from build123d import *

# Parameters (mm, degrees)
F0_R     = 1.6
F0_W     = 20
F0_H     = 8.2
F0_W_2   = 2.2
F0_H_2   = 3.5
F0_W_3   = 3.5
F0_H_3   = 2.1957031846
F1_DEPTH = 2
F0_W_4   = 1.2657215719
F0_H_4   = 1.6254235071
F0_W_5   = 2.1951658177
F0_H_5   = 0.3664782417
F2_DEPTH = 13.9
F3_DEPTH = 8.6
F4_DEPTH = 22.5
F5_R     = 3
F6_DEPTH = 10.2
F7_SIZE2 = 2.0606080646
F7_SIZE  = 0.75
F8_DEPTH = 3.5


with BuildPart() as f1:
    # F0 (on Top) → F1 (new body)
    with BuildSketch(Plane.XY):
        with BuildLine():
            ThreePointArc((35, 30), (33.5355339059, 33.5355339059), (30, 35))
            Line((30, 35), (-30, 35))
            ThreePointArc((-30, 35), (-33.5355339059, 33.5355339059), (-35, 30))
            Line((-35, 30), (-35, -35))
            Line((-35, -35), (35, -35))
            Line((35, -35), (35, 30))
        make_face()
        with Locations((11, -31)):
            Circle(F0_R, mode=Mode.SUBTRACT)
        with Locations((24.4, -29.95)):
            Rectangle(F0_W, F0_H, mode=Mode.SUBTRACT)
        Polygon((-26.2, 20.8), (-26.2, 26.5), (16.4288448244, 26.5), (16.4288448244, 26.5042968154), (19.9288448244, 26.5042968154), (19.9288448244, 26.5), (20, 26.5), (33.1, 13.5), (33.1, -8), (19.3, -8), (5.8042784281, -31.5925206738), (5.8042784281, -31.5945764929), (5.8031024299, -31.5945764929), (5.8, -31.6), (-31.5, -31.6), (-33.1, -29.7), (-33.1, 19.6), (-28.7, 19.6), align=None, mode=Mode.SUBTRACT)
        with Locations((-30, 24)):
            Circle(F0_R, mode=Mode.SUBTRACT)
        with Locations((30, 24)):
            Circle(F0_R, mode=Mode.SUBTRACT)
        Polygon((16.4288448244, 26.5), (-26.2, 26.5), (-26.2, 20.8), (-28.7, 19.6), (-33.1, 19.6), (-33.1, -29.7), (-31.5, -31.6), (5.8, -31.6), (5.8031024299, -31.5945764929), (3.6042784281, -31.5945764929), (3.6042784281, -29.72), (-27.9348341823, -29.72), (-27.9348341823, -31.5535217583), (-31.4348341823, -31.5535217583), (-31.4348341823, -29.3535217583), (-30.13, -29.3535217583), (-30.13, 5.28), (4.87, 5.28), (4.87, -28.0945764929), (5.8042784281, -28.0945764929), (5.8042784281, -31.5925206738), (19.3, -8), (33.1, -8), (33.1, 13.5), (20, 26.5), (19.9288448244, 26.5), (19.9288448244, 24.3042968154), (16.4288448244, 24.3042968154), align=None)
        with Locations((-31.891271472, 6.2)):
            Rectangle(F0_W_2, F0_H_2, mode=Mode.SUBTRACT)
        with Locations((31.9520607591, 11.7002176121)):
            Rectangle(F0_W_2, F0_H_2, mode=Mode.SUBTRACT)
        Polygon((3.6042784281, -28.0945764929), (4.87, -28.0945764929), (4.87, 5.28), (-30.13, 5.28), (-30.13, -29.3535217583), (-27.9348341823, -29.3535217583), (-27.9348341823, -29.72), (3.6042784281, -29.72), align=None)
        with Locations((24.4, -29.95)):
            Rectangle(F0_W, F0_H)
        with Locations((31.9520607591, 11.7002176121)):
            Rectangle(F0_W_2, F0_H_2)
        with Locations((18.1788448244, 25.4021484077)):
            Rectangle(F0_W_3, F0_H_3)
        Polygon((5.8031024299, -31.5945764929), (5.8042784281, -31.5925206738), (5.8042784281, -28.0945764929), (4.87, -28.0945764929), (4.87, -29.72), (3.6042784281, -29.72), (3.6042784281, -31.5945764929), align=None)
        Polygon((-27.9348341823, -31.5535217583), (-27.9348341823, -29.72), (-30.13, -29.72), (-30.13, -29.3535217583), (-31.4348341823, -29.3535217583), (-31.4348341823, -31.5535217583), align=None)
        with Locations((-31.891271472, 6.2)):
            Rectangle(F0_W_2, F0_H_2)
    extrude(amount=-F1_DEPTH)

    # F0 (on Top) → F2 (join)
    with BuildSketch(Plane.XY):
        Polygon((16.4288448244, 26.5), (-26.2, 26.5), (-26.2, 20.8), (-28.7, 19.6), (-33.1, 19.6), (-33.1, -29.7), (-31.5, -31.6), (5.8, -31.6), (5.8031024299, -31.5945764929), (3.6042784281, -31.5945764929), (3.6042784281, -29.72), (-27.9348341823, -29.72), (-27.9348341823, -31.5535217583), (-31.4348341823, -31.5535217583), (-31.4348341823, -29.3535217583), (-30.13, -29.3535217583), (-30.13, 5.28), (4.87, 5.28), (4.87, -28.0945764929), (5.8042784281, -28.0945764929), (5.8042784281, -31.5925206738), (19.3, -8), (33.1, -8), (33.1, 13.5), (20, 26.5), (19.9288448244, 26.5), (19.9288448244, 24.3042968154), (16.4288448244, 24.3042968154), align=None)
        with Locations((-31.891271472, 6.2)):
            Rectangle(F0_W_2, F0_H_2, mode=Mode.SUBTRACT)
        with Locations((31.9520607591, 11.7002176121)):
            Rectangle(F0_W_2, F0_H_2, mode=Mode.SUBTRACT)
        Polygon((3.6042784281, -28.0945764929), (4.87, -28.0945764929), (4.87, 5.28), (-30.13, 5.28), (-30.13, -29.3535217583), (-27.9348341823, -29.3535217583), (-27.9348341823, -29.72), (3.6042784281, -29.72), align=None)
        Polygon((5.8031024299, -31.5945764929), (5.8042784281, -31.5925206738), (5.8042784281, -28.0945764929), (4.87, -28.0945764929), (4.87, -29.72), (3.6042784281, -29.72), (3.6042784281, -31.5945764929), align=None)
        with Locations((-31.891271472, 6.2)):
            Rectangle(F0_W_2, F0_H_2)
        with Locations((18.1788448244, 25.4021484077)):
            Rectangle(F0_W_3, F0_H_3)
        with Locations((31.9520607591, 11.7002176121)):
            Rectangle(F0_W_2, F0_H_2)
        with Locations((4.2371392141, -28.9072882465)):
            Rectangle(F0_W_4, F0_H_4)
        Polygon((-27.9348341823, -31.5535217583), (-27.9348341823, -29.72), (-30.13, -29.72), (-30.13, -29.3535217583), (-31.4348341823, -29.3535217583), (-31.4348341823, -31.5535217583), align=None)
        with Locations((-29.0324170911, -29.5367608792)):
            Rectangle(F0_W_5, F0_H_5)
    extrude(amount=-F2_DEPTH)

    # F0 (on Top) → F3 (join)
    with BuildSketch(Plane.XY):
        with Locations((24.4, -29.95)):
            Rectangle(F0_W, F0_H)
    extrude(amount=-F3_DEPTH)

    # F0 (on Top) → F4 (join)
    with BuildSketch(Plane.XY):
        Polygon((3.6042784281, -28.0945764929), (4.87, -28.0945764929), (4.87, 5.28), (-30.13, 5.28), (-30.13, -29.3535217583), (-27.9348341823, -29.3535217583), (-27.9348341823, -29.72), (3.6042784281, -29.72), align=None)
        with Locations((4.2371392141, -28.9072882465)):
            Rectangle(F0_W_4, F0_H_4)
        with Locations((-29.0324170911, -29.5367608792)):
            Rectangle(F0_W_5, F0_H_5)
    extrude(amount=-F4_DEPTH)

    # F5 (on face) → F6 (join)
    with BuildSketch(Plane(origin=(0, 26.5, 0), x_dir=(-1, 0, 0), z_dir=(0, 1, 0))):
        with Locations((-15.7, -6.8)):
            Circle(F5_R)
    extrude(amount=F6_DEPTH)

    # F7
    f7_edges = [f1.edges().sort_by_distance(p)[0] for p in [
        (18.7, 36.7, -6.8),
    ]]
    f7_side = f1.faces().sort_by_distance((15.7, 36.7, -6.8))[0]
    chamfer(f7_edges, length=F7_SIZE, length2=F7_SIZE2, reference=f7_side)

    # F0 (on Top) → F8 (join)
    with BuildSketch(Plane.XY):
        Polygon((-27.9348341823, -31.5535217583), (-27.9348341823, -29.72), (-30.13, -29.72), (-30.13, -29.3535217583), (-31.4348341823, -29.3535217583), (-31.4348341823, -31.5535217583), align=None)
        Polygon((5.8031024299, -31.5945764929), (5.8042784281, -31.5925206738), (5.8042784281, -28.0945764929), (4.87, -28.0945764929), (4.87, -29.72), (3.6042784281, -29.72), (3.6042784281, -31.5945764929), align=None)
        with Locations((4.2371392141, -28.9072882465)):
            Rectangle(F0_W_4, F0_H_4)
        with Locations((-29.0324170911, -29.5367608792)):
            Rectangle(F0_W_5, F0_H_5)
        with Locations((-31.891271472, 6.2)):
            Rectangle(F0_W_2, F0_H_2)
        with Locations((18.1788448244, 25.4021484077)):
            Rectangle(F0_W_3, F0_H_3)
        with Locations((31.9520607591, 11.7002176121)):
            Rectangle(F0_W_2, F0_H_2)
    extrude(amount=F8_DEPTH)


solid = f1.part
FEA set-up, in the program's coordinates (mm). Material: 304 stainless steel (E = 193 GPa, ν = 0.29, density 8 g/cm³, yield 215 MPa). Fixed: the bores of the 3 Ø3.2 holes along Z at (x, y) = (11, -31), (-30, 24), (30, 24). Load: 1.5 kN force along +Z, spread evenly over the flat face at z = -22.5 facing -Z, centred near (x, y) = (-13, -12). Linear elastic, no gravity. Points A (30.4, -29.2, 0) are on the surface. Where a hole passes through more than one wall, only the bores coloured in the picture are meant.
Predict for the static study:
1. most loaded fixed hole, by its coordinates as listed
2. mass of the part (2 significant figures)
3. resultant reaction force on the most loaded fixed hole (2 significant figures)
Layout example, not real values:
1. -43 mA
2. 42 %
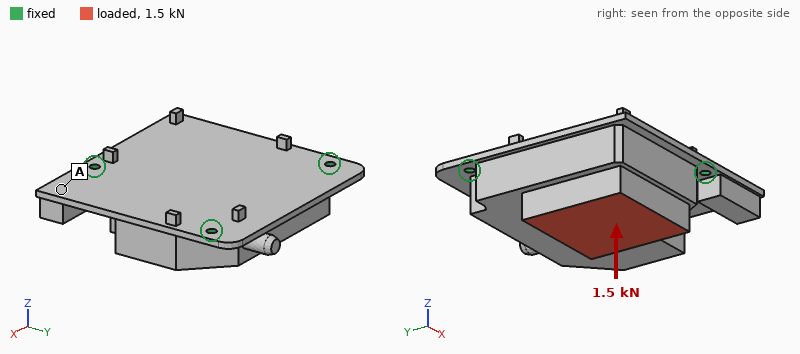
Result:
1. (11, -31)
2. 480 g
3. 1.2 kN
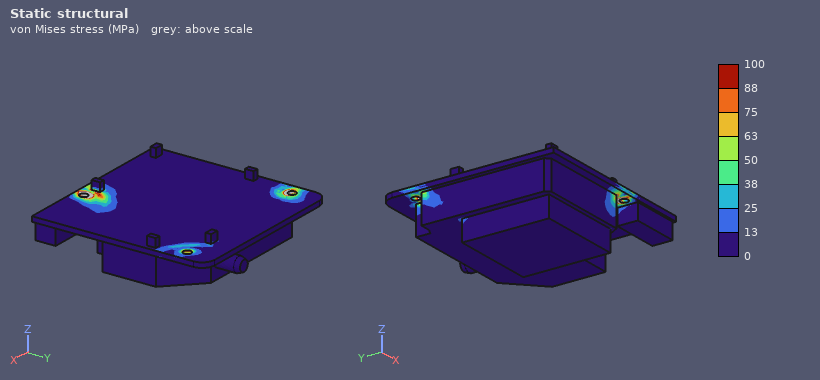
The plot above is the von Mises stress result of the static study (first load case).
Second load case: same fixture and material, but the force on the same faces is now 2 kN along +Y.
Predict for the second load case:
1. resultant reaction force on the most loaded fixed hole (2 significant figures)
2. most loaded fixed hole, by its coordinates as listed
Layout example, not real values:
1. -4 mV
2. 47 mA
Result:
1. 1.2 kN
2. (11, -31)
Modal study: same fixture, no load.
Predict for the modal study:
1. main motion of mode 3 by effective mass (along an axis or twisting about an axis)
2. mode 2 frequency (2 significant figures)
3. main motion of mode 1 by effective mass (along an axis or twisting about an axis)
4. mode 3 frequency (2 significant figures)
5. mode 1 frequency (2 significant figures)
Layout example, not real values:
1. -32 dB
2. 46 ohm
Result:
1. along Z
2. 3600 Hz
3. along Z
4. 4400 Hz
5. 3000 Hz
